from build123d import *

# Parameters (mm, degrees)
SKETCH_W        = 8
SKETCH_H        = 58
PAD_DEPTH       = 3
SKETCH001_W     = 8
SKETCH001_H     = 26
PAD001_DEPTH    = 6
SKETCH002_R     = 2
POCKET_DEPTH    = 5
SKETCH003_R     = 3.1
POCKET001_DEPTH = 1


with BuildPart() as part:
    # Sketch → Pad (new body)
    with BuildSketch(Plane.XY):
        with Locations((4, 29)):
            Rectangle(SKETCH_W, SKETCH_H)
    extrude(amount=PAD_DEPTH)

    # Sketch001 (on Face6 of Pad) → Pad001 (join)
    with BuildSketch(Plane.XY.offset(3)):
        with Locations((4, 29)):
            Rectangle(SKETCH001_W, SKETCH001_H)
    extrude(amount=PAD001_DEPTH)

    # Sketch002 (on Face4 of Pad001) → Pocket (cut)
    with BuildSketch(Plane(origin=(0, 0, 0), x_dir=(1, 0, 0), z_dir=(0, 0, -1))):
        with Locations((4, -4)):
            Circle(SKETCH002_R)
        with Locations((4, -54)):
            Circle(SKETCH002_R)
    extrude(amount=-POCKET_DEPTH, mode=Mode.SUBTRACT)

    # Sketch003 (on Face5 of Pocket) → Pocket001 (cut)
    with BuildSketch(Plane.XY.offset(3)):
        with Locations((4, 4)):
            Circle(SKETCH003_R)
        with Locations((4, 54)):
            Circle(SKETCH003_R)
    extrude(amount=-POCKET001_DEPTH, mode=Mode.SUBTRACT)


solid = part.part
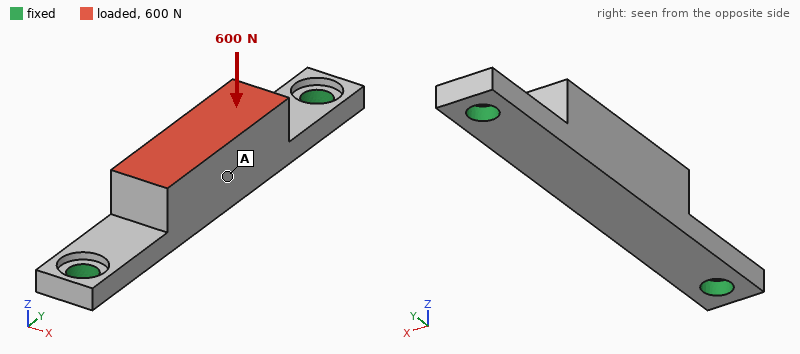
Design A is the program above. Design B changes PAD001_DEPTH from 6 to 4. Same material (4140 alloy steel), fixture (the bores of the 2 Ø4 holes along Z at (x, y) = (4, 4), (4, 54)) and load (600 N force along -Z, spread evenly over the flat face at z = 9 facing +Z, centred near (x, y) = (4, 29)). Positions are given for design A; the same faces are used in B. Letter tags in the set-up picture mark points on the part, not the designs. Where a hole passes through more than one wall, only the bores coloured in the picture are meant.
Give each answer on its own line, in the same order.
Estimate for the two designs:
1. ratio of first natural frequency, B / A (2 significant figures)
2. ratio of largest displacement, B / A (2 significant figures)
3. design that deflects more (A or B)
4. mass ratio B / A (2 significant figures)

1.1
1.2
B
0.84
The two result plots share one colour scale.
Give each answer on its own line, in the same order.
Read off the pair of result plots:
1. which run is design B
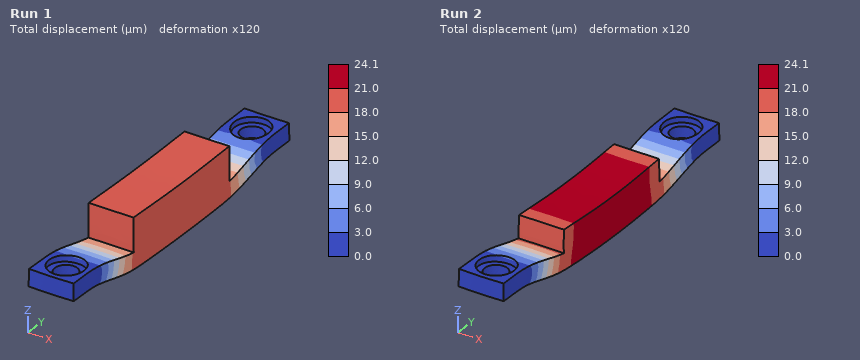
Run 2
